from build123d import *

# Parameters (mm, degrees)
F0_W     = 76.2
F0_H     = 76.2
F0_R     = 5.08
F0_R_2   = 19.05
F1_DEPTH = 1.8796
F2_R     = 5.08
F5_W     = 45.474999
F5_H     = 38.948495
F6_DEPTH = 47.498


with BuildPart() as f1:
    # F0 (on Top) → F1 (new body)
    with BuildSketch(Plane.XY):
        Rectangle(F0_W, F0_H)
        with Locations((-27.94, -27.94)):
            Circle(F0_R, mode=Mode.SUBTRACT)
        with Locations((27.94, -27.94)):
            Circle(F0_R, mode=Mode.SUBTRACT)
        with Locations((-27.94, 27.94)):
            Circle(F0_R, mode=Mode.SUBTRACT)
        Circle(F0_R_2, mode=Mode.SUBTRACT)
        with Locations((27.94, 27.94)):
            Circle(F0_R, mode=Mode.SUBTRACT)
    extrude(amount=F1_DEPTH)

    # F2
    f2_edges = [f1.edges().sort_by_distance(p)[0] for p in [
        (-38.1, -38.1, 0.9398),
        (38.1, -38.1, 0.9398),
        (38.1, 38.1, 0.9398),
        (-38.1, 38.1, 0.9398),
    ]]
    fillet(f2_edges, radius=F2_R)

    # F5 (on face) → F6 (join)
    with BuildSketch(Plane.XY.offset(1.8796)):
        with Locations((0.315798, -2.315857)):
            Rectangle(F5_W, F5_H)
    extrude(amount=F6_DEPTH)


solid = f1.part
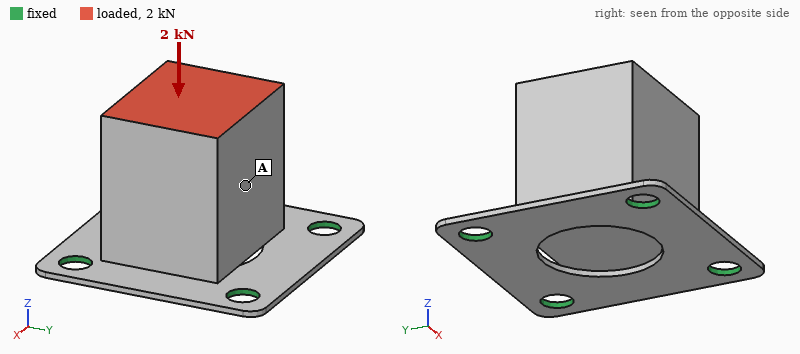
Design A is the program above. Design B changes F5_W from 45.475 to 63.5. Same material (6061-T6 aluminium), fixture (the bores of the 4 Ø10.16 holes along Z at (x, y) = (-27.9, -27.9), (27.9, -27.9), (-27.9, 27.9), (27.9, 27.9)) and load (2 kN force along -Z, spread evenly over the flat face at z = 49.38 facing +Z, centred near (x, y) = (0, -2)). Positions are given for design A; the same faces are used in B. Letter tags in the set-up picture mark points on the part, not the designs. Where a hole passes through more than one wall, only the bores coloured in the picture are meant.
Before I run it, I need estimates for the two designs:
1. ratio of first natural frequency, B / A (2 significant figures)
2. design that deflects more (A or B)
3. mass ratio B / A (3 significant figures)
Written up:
1.2
A
1.36
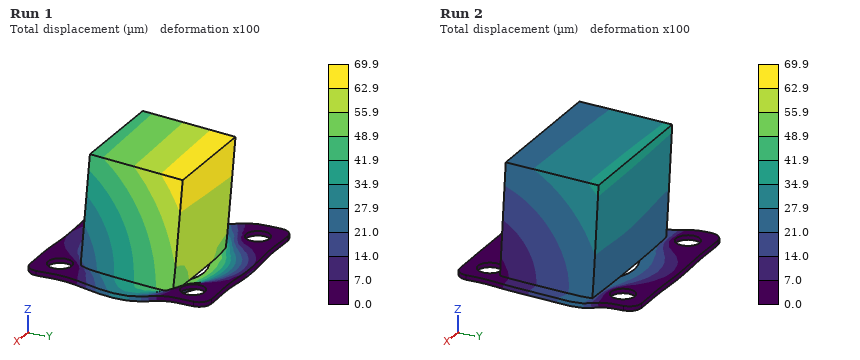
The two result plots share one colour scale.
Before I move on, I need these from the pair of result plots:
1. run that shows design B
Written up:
Run 2
